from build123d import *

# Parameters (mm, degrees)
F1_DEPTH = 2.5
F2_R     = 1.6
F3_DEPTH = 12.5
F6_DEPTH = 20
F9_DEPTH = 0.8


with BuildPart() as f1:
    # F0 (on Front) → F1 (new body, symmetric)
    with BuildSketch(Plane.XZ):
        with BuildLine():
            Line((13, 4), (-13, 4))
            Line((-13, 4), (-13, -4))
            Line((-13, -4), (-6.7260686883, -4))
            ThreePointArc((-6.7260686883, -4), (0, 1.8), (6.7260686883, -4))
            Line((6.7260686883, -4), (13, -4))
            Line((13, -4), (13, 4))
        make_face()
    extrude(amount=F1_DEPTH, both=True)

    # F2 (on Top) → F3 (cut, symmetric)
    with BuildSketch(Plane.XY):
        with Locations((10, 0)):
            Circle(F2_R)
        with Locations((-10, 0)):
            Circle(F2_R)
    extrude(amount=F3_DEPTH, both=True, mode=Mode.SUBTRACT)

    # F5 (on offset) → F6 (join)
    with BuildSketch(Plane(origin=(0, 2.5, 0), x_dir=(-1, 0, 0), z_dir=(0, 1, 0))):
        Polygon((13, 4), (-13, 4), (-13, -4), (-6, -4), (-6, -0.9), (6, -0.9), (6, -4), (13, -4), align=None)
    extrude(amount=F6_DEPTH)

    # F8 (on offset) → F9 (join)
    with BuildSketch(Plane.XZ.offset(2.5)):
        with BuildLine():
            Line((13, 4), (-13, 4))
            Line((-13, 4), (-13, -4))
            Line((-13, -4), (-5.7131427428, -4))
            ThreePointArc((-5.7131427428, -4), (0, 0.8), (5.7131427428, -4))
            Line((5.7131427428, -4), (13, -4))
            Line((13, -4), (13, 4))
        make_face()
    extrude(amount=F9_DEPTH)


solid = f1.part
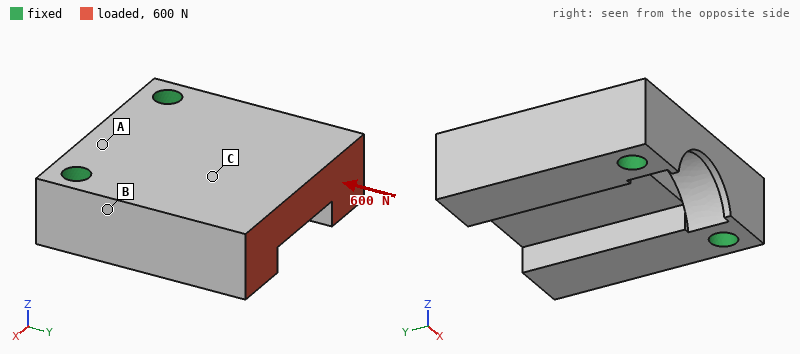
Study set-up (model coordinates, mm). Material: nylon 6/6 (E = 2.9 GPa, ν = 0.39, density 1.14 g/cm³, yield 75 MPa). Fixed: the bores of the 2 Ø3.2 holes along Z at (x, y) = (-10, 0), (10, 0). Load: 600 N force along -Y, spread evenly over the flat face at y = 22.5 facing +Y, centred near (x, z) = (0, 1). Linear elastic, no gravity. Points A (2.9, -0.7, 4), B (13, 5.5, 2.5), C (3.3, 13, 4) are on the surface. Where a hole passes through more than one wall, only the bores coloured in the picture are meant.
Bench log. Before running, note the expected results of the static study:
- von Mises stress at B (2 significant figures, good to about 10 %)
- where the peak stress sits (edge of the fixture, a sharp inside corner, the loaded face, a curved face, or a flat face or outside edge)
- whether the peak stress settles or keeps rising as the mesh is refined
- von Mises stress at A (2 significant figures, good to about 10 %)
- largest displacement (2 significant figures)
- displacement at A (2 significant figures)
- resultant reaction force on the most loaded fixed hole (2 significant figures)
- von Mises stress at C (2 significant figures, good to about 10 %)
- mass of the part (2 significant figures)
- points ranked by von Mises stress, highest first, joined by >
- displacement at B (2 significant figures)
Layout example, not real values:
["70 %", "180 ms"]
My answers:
["4.6 MPa", "edge of the fixture", "keeps rising", "1.2 MPa", "38 µm", "14 µm", "310 N", "3.1 MPa", "4.7 g", "B > C > A", "10.0 µm"]
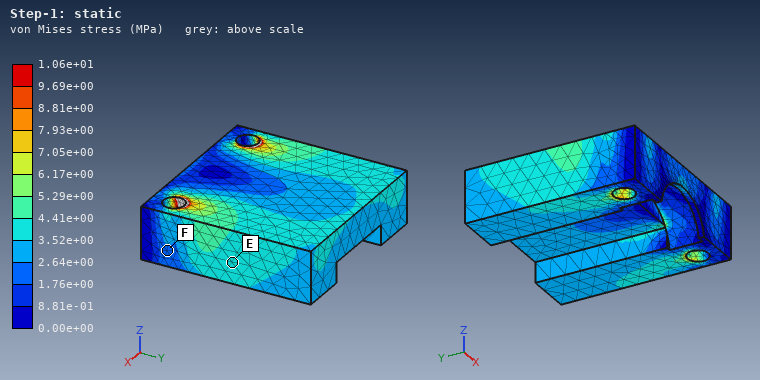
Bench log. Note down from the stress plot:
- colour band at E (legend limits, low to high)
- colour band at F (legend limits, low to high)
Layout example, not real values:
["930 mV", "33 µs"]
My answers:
["3.52e+00 to 4.41e+00 MPa", "1.76e+00 to 2.64e+00 MPa"]
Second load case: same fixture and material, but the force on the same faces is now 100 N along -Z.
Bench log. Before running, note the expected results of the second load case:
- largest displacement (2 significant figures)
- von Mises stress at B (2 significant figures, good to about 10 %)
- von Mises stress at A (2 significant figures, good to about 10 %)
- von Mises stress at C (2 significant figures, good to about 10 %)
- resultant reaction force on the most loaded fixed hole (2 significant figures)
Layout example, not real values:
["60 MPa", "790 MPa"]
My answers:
["0.20 mm", "5.2 MPa", "2.1 MPa", "3.7 MPa", "52 N"]
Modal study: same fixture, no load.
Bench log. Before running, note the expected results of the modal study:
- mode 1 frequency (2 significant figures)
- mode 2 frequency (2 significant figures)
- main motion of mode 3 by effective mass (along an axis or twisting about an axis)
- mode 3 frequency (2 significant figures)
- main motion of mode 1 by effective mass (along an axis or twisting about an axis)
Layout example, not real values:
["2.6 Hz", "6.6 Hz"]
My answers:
["3400 Hz", "5500 Hz", "along X", "7800 Hz", "along Z"]
